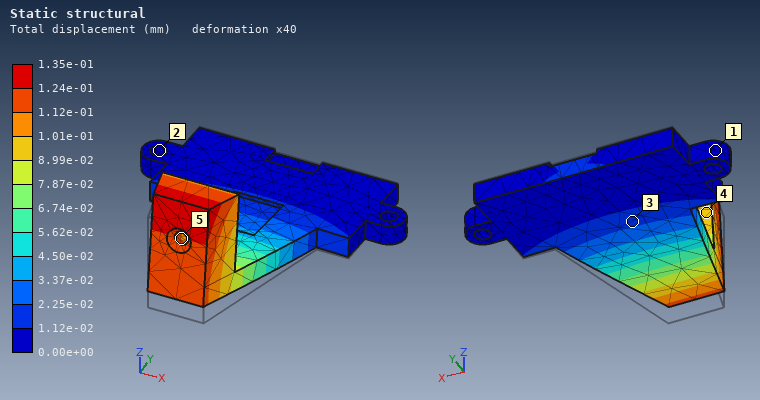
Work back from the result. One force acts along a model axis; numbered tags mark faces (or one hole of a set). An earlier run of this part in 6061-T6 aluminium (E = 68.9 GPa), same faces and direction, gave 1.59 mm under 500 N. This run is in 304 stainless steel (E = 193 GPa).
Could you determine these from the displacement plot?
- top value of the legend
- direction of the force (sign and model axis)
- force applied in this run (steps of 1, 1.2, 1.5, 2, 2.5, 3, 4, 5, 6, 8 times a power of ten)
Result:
1.35e-01 mm
+Z
120 N
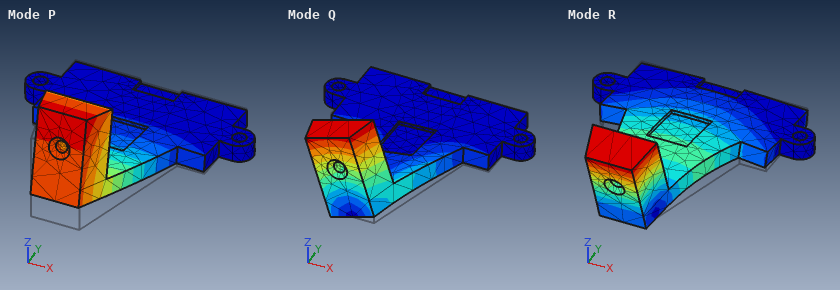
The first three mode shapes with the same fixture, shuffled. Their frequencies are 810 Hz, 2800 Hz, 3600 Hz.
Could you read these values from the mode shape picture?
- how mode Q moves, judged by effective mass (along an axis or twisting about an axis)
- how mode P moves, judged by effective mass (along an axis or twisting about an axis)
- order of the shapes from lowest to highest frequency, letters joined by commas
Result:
along X
along Z
P, Q, R
